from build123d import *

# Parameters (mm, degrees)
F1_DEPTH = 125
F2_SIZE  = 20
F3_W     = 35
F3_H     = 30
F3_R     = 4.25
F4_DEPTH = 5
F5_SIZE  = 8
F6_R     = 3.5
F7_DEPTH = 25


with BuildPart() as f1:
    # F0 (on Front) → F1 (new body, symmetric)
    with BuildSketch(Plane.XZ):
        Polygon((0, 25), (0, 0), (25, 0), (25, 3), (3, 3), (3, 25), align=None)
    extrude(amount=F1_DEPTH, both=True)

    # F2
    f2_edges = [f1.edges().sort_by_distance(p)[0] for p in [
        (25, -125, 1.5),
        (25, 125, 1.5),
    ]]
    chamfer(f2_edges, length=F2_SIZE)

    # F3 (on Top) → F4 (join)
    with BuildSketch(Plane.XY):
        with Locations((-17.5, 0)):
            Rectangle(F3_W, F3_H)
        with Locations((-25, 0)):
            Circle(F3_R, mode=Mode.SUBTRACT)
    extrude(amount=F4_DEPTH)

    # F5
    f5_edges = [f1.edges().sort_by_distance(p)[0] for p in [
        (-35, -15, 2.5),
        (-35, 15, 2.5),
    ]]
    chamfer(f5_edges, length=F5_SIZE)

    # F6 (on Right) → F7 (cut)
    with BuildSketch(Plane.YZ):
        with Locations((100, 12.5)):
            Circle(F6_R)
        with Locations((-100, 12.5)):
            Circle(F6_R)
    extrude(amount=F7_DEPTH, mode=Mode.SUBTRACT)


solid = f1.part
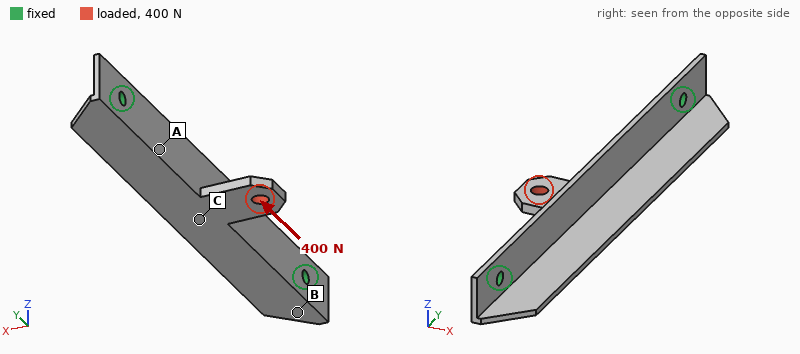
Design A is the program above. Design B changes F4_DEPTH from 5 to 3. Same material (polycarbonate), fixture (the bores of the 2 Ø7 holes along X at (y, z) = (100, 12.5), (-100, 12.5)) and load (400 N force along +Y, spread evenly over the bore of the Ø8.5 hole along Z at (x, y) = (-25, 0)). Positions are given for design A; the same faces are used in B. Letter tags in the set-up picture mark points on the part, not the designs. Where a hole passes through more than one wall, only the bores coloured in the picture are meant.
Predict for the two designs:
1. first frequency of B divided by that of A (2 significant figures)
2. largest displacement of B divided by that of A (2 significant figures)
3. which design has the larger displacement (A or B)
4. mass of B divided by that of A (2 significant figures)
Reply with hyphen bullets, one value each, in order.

- 1.1
- 1.1
- B
- 0.95
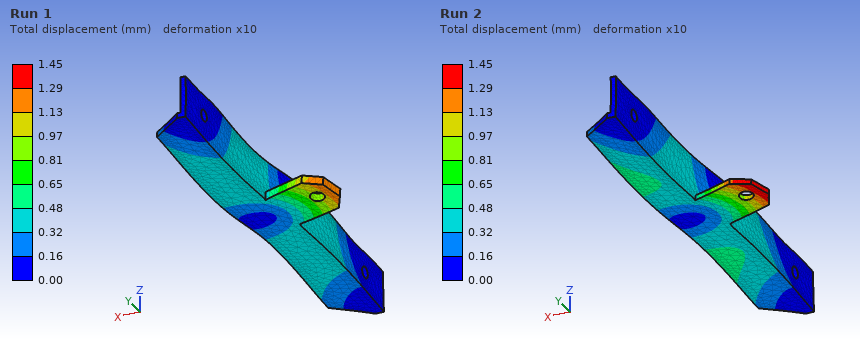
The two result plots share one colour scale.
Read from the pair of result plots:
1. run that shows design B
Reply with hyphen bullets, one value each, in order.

- Run 2
